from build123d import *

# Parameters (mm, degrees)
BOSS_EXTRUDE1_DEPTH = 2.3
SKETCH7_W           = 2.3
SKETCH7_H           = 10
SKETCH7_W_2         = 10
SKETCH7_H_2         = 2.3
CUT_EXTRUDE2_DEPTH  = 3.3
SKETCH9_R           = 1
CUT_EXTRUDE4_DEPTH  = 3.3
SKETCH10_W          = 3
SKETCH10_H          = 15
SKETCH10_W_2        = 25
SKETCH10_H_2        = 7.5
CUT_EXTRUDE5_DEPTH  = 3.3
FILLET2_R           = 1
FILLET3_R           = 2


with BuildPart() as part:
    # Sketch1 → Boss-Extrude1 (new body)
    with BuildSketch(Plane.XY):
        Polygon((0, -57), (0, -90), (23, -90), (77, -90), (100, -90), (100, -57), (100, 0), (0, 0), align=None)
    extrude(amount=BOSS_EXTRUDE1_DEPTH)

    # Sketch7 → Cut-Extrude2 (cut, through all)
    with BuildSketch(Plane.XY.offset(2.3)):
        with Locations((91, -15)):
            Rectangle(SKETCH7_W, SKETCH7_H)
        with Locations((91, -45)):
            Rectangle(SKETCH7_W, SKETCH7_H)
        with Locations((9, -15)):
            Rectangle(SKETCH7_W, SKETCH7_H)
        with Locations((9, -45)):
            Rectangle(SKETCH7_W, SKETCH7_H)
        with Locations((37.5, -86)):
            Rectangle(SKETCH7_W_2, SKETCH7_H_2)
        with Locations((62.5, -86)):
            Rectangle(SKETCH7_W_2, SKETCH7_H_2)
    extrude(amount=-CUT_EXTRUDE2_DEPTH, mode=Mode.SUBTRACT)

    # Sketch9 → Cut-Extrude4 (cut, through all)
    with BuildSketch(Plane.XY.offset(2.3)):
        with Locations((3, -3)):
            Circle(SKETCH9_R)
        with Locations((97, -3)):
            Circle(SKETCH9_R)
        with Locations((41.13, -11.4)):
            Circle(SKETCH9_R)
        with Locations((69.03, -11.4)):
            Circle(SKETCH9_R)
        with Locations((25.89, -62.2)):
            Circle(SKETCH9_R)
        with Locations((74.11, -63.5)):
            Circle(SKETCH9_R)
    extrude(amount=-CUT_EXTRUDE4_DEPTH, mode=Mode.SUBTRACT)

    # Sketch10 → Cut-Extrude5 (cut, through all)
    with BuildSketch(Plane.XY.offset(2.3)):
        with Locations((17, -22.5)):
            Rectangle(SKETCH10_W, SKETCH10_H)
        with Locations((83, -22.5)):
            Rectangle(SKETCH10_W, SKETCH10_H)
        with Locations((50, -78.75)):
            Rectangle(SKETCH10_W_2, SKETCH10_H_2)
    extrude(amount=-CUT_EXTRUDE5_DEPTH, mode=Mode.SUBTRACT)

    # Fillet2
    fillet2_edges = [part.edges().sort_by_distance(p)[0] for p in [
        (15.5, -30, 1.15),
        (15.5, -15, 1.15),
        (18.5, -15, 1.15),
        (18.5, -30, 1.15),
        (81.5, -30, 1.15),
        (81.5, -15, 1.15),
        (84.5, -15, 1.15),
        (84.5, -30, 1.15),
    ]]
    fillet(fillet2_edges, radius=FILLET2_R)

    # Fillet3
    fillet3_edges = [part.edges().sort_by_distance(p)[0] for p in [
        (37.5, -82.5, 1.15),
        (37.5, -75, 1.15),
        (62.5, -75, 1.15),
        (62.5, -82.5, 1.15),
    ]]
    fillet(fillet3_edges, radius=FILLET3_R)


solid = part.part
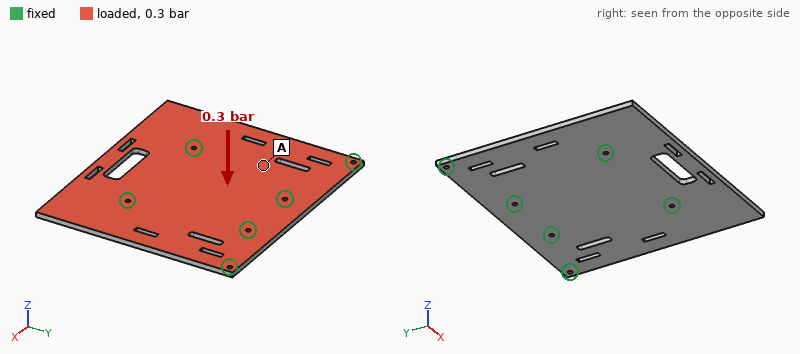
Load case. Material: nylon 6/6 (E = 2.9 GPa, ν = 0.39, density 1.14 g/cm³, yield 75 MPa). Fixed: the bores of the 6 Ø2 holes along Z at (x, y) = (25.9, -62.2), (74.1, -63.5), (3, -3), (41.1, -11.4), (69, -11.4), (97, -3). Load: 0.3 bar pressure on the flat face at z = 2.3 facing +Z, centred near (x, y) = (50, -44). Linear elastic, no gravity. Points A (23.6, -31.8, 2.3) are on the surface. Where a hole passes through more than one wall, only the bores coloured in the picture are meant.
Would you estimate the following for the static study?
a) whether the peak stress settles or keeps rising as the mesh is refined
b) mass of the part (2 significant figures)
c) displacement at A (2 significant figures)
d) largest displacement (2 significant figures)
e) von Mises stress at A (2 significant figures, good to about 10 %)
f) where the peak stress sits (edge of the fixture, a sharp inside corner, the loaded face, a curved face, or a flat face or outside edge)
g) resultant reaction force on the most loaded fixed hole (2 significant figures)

keeps rising
22 g
0.32 mm
1.4 mm
3.7 MPa
edge of the fixture
81 N
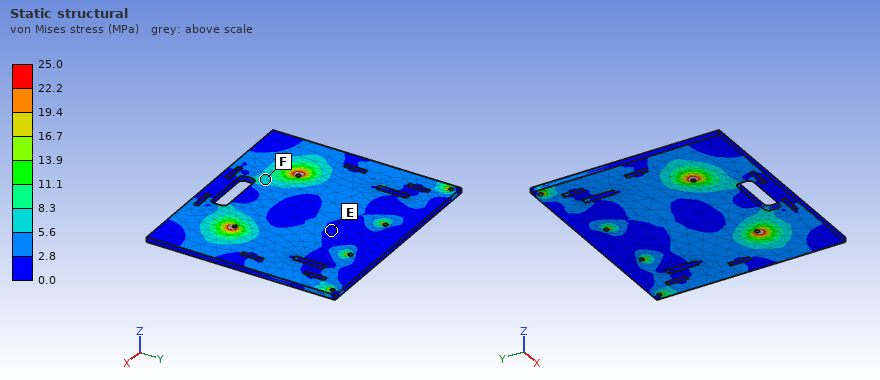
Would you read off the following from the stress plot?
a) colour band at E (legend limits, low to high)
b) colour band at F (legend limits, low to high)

0.0 to 2.8 MPa
5.6 to 8.3 MPa
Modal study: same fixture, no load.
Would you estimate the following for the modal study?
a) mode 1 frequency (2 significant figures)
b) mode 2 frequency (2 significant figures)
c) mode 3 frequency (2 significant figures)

580 Hz
630 Hz
670 Hz
